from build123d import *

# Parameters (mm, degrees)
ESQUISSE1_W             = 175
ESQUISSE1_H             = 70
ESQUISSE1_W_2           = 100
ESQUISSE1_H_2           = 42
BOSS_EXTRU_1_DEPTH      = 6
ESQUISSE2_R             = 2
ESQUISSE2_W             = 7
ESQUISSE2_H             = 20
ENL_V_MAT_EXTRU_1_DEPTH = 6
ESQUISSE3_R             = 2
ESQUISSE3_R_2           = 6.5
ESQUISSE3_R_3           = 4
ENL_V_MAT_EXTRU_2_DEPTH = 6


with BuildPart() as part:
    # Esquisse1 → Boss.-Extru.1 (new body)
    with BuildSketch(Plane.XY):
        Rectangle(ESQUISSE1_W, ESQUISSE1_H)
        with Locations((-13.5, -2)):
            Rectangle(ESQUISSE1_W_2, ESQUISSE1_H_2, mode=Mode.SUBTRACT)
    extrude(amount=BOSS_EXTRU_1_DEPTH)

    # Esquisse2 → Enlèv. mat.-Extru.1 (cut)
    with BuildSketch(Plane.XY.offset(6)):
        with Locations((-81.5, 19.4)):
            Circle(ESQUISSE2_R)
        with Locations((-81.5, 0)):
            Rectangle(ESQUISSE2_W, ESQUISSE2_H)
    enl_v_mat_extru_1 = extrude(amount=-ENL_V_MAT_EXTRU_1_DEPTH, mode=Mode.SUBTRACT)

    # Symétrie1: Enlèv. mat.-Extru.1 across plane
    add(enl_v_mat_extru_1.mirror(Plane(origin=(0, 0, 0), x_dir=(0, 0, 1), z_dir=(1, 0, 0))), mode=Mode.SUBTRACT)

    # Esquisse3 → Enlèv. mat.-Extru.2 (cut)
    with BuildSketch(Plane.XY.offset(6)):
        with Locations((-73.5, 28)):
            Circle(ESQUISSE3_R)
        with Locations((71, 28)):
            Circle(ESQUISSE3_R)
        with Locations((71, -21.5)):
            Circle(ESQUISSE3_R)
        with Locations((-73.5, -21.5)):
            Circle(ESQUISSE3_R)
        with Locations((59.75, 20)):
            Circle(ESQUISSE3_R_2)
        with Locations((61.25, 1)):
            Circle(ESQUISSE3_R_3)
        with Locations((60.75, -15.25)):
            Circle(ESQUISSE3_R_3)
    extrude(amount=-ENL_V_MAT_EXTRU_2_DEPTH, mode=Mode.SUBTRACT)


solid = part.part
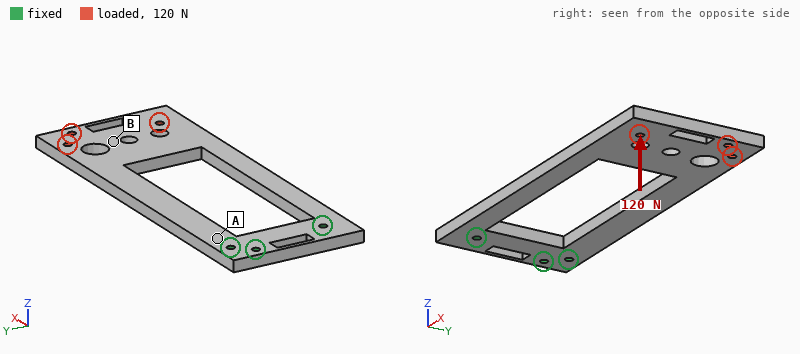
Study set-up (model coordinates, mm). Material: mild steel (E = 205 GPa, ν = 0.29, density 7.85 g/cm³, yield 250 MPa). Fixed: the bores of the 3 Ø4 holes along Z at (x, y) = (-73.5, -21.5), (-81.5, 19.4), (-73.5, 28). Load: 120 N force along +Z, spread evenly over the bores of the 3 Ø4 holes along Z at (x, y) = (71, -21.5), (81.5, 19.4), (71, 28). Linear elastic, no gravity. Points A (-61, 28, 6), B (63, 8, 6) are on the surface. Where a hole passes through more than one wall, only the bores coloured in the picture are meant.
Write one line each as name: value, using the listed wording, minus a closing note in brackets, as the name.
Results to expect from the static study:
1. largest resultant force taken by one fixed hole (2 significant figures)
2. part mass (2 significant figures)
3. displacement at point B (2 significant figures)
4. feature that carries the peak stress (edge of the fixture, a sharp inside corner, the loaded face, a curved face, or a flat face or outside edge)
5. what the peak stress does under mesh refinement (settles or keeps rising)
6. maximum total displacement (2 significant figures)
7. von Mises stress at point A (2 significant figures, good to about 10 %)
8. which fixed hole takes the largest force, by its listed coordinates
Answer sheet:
largest resultant force taken by one fixed hole: 310 N
part mass: 350 g
displacement at point B: 1.1 mm
feature that carries the peak stress: edge of the fixture
what the peak stress does under mesh refinement: keeps rising
maximum total displacement: 1.4 mm
von Mises stress at point A: 93 MPa
which fixed hole takes the largest force, by its listed coordinates: (-73.5, 28)
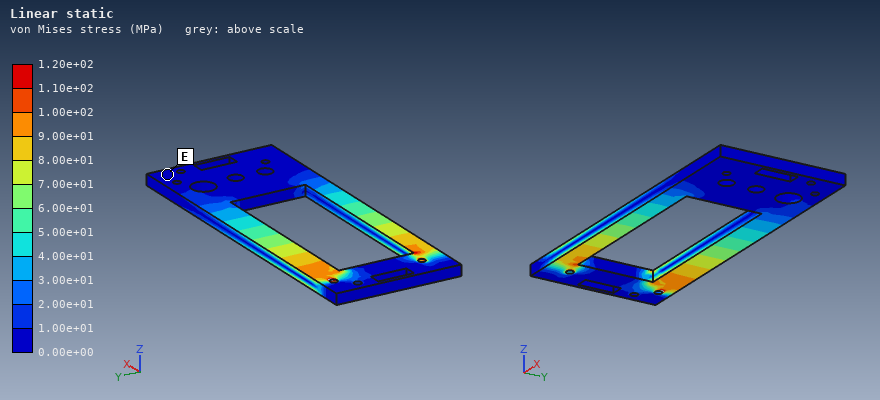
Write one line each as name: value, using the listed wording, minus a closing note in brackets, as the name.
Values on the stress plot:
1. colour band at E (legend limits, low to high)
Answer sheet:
colour band at E: 0.00e+00 to 1.00e+01 MPa
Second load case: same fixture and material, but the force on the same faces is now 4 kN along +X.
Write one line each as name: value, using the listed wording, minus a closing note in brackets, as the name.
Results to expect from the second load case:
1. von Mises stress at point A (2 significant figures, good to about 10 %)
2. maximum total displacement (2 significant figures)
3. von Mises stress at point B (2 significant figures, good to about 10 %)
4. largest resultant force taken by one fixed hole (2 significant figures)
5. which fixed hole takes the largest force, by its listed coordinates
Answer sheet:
von Mises stress at point A: 29 MPa
maximum total displacement: 21 µm
von Mises stress at point B: 12 MPa
largest resultant force taken by one fixed hole: 2.1 kN
which fixed hole takes the largest force, by its listed coordinates: (-73.5, 28)
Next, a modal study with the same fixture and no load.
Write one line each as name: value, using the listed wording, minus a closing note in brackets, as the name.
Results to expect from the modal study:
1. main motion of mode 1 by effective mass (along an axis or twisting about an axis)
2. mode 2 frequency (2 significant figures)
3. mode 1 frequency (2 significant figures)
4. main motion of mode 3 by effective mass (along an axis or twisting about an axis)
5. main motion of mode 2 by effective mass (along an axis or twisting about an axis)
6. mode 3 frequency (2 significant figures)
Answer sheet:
main motion of mode 1 by effective mass: along Z
mode 2 frequency: 610 Hz
mode 1 frequency: 140 Hz
main motion of mode 3 by effective mass: along Y
main motion of mode 2 by effective mass: twisting about X
mode 3 frequency: 700 Hz
